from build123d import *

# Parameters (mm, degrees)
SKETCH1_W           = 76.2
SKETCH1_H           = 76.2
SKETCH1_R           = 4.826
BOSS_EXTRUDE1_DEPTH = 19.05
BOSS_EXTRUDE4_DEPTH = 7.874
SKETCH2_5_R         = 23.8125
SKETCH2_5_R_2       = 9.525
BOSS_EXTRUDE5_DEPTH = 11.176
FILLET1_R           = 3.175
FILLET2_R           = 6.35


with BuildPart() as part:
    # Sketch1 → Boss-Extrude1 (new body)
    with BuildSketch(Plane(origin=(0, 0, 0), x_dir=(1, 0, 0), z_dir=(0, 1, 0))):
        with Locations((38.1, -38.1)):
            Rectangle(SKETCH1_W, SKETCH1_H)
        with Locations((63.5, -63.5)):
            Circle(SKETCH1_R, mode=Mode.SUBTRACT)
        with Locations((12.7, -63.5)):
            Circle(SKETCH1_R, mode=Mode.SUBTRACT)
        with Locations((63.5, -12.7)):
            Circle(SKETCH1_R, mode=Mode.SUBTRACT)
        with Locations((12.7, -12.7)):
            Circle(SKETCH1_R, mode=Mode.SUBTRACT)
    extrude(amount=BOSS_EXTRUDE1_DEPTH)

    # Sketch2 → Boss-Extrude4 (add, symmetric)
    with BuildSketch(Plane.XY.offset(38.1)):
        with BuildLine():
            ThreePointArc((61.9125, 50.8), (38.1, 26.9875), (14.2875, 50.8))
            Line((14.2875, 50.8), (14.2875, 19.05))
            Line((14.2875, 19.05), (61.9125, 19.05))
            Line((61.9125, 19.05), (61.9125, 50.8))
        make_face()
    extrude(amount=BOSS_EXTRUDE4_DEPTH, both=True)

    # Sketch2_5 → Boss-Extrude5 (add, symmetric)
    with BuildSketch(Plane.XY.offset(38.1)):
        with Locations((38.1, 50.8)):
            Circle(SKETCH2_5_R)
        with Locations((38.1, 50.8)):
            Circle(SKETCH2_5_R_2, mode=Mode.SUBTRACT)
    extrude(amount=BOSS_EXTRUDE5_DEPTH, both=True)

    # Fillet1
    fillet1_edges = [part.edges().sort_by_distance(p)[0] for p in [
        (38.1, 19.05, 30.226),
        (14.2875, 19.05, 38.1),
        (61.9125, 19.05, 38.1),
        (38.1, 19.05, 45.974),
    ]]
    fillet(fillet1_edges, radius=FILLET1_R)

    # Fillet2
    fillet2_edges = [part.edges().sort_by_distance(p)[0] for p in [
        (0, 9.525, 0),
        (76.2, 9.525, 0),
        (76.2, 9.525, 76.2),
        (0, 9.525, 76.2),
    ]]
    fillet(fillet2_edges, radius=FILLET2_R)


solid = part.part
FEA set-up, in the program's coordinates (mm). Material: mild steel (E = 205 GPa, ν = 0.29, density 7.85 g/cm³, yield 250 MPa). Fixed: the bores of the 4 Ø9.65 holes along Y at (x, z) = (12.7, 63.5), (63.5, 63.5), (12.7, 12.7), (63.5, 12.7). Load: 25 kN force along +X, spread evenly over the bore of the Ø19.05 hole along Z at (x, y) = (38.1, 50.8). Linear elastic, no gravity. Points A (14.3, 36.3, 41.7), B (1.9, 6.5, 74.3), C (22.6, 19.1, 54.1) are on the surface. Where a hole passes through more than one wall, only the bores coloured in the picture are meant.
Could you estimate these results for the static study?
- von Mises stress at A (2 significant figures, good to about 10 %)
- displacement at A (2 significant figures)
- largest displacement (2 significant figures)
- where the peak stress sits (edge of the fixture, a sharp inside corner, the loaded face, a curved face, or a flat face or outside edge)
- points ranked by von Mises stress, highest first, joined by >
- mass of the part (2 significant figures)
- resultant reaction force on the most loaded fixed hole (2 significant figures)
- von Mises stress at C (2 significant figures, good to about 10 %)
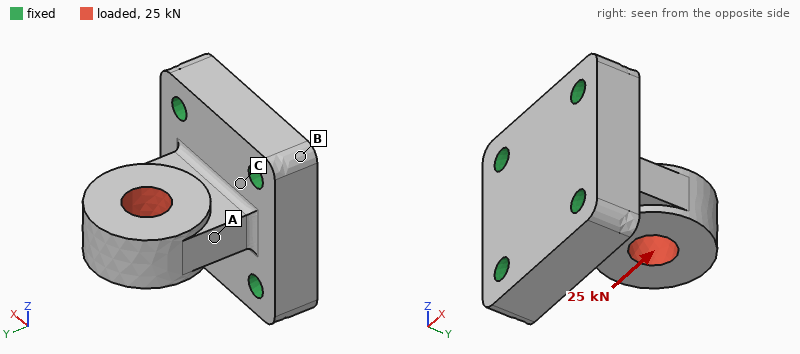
78 MPa
29 µm
65 µm
a curved face
A > C > B
1.2 kg
12 kN
45 MPa
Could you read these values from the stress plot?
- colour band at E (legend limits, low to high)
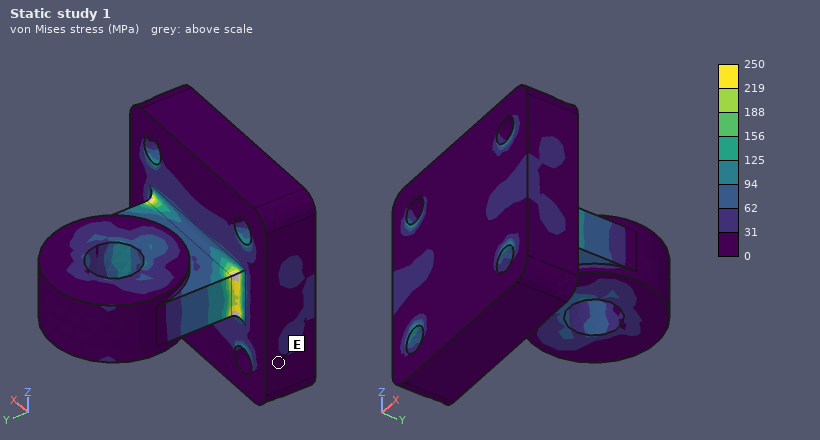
0 to 31 MPa
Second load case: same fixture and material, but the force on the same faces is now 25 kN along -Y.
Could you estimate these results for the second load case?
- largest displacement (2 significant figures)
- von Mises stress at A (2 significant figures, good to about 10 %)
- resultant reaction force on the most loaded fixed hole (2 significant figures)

14 µm
29 MPa
6.4 kN
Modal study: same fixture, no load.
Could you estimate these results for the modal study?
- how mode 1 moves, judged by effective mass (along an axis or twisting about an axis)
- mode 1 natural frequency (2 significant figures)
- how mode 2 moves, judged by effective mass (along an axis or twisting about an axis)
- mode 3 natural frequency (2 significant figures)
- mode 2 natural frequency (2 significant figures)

along Z
3800 Hz
along X
9900 Hz
6700 Hz
